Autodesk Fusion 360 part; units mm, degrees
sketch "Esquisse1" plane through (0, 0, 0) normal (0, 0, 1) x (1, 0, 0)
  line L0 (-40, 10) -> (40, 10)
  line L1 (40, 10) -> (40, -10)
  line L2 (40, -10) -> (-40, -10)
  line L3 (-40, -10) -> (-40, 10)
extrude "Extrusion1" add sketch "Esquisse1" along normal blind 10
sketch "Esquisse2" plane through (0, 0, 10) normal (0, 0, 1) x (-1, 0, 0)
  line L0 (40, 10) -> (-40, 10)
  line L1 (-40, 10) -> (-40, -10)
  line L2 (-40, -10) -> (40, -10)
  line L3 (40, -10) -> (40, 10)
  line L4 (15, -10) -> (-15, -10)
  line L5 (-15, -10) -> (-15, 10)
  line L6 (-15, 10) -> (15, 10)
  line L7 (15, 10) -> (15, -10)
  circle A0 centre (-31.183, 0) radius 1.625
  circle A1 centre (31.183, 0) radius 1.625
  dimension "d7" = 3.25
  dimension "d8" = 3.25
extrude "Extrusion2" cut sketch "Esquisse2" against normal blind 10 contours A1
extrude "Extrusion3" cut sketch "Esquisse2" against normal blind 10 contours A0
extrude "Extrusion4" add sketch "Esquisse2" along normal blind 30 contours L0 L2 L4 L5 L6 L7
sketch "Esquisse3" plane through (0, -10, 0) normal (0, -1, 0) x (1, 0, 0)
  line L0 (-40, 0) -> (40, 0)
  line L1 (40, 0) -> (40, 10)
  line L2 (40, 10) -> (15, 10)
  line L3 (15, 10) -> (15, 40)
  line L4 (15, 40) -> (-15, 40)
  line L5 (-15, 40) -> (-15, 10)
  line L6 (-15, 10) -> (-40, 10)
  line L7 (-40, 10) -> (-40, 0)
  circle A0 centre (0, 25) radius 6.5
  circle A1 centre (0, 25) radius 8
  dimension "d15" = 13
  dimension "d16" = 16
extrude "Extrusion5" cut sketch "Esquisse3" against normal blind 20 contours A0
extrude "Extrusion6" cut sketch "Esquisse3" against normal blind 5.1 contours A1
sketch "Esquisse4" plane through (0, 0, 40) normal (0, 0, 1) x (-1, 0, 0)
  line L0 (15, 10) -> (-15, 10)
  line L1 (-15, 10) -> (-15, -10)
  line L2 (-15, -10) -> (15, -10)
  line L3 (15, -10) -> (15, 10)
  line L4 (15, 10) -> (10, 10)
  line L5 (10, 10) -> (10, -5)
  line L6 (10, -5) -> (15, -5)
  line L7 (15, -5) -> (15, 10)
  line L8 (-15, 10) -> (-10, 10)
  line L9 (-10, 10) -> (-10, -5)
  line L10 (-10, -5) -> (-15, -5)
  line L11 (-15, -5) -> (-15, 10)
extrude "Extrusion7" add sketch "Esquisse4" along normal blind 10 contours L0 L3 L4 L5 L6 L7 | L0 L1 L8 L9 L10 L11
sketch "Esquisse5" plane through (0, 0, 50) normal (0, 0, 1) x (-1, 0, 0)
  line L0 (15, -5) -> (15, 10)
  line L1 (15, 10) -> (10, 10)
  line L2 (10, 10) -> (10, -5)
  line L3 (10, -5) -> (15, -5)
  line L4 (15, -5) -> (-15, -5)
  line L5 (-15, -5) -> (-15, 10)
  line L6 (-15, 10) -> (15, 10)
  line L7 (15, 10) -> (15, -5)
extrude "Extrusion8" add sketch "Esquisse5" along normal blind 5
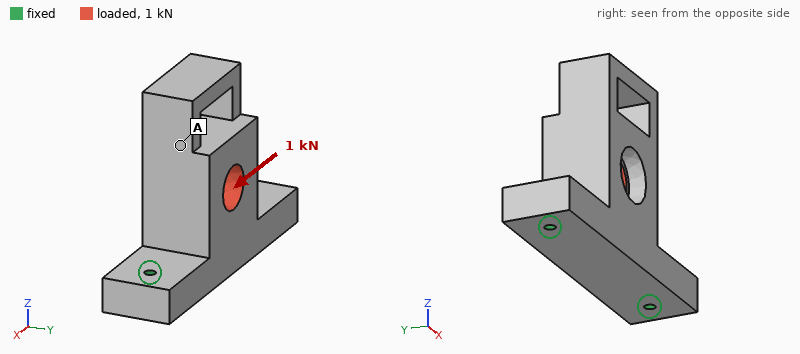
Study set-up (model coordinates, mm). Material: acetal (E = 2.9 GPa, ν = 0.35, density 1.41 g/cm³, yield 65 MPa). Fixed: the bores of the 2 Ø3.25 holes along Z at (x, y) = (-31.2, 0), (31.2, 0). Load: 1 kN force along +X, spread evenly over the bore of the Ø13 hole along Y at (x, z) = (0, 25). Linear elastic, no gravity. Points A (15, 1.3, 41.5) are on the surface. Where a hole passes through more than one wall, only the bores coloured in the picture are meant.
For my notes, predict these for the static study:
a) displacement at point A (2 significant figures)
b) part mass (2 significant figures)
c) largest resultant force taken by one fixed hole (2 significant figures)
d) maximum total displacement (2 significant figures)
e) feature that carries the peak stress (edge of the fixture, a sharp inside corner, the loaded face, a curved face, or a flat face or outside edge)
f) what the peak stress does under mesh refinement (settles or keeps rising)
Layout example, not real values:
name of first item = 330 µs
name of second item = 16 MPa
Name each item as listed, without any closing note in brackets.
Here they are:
displacement at point A = 0.30 mm
part mass = 49 g
largest resultant force taken by one fixed hole = 640 N
maximum total displacement = 0.39 mm
feature that carries the peak stress = edge of the fixture
what the peak stress does under mesh refinement = keeps rising
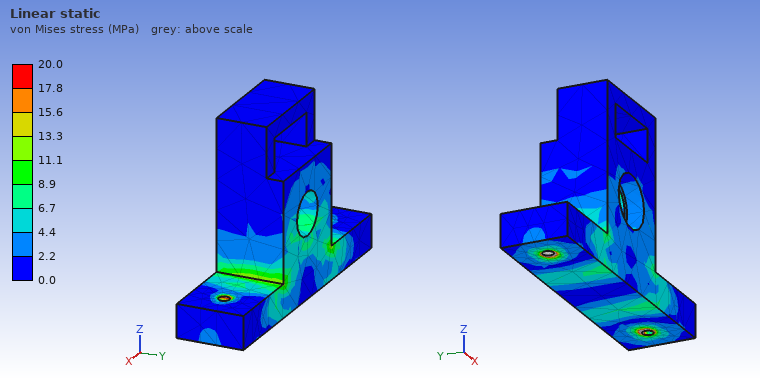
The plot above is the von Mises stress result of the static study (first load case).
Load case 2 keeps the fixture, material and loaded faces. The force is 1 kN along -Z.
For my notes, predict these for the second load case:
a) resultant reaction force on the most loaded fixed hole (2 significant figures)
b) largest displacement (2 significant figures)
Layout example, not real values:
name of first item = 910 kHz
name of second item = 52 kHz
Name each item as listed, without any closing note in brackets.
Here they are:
resultant reaction force on the most loaded fixed hole = 530 N
largest displacement = 0.36 mm
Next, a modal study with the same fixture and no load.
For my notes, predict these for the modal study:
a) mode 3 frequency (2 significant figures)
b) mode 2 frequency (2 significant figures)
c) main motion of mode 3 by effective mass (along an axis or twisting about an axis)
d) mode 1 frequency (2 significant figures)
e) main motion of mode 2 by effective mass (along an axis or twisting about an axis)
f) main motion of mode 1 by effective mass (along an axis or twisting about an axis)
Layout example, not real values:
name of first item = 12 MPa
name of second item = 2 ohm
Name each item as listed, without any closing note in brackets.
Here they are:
mode 3 frequency = 2000 Hz
mode 2 frequency = 1500 Hz
main motion of mode 3 by effective mass = along Z
mode 1 frequency = 680 Hz
main motion of mode 2 by effective mass = along X
main motion of mode 1 by effective mass = along Y
